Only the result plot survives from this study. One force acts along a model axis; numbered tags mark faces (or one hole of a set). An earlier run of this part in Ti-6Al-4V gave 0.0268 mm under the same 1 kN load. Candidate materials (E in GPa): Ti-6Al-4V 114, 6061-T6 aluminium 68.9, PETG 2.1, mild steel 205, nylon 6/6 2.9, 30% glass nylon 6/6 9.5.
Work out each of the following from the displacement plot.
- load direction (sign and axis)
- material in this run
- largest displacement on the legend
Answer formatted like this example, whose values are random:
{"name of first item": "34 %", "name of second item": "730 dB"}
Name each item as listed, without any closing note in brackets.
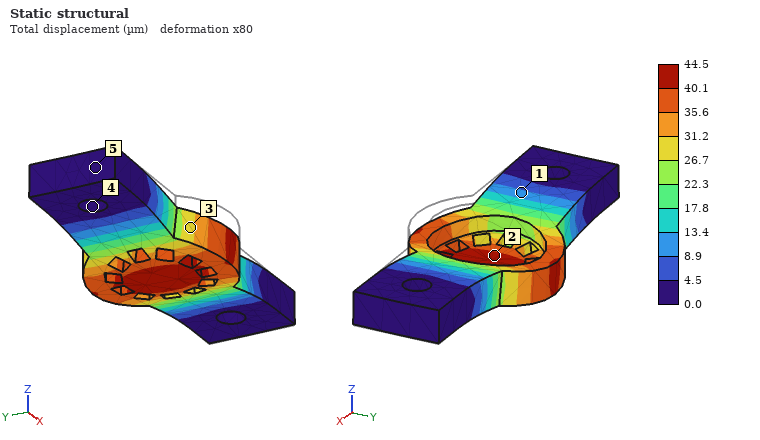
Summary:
{"load direction": "-Z", "material in this run": "6061-T6 aluminium", "largest displacement on the legend": "44.5 µm"}
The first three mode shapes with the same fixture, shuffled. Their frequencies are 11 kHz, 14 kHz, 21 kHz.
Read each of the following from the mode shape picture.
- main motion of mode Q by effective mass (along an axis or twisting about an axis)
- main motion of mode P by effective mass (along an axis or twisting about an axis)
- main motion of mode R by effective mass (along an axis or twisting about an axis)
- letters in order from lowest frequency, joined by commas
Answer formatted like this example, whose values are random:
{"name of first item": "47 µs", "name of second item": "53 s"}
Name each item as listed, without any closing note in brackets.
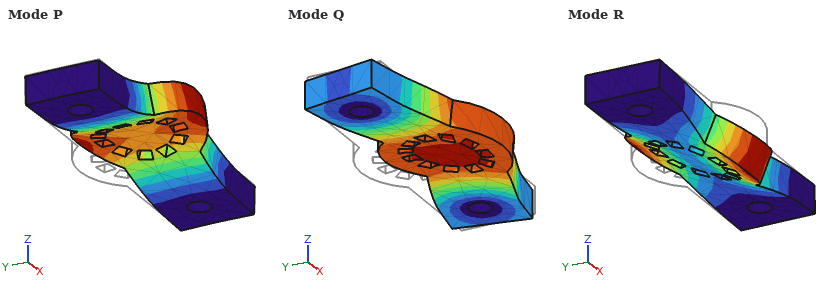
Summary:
{"main motion of mode Q by effective mass": "along Y", "main motion of mode P by effective mass": "along Z", "main motion of mode R by effective mass": "twisting about X", "letters in order from lowest frequency, joined by commas": "P, R, Q"}
